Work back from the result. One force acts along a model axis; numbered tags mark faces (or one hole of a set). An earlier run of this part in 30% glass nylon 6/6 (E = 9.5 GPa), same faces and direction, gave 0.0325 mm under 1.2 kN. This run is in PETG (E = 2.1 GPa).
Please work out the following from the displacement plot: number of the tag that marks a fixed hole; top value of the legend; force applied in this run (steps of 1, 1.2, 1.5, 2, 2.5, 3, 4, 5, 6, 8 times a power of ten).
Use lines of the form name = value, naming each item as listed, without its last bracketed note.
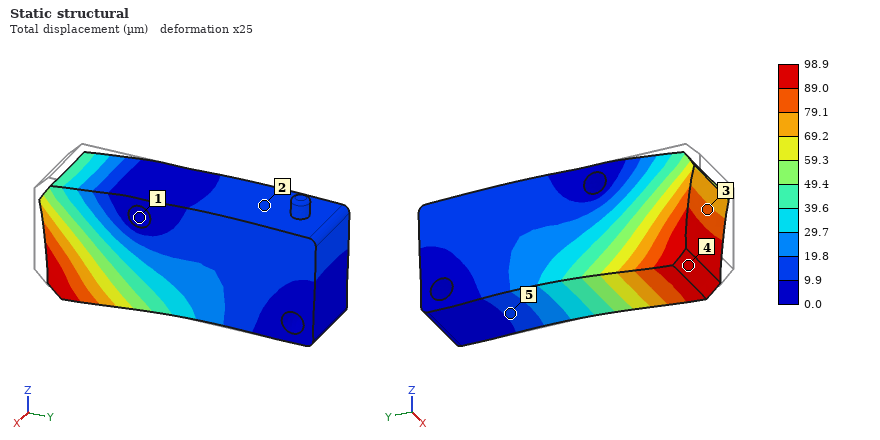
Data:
number of the tag that marks a fixed hole = 1
top value of the legend = 98.9 µm
force applied in this run = 800 N
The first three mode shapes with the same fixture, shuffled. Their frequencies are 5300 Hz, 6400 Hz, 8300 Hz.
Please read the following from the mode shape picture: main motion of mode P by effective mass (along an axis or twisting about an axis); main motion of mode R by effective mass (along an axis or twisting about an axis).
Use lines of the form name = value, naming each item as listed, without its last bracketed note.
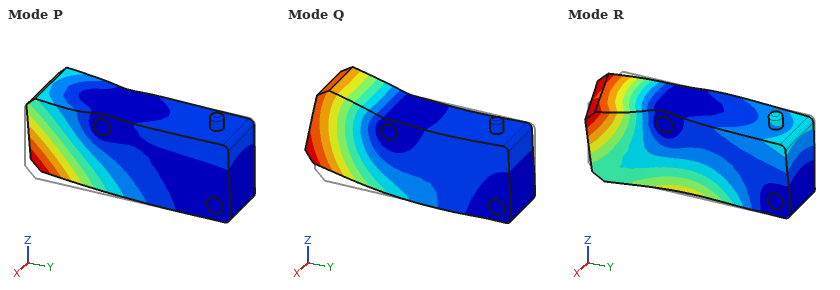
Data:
main motion of mode P by effective mass = along X
main motion of mode R by effective mass = twisting about Y
